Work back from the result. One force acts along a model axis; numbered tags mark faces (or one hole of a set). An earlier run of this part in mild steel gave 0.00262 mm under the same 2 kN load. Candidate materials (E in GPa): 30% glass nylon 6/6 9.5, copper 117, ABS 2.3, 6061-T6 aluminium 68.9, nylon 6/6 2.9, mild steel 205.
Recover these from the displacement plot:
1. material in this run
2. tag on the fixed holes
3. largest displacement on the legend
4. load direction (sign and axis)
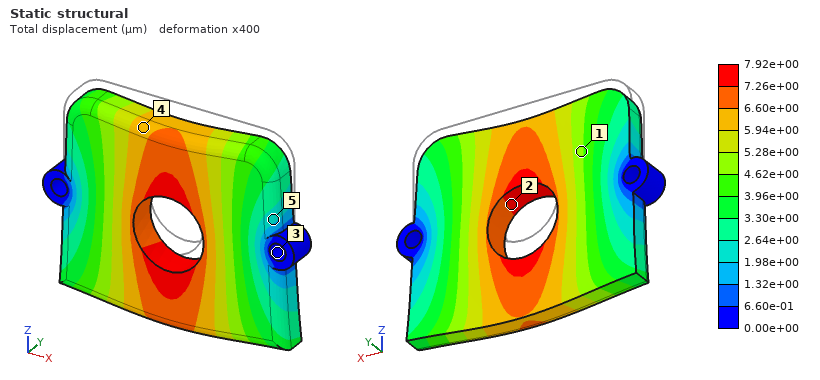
6061-T6 aluminium
3
7.92e+00 µm
-Z
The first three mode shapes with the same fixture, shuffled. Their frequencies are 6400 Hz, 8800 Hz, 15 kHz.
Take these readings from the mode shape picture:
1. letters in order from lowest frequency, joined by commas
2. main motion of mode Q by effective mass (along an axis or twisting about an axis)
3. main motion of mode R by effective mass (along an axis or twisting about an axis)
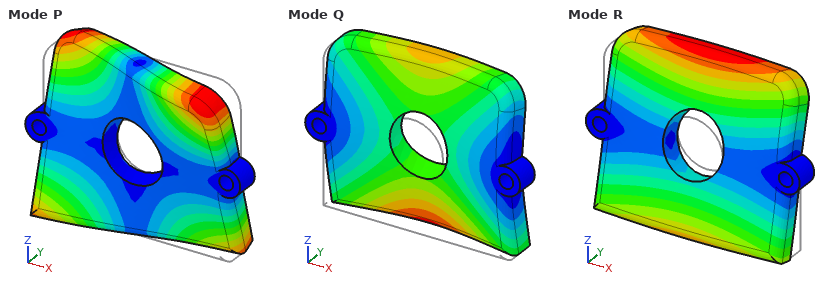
R, Q, P
along Y
twisting about X
